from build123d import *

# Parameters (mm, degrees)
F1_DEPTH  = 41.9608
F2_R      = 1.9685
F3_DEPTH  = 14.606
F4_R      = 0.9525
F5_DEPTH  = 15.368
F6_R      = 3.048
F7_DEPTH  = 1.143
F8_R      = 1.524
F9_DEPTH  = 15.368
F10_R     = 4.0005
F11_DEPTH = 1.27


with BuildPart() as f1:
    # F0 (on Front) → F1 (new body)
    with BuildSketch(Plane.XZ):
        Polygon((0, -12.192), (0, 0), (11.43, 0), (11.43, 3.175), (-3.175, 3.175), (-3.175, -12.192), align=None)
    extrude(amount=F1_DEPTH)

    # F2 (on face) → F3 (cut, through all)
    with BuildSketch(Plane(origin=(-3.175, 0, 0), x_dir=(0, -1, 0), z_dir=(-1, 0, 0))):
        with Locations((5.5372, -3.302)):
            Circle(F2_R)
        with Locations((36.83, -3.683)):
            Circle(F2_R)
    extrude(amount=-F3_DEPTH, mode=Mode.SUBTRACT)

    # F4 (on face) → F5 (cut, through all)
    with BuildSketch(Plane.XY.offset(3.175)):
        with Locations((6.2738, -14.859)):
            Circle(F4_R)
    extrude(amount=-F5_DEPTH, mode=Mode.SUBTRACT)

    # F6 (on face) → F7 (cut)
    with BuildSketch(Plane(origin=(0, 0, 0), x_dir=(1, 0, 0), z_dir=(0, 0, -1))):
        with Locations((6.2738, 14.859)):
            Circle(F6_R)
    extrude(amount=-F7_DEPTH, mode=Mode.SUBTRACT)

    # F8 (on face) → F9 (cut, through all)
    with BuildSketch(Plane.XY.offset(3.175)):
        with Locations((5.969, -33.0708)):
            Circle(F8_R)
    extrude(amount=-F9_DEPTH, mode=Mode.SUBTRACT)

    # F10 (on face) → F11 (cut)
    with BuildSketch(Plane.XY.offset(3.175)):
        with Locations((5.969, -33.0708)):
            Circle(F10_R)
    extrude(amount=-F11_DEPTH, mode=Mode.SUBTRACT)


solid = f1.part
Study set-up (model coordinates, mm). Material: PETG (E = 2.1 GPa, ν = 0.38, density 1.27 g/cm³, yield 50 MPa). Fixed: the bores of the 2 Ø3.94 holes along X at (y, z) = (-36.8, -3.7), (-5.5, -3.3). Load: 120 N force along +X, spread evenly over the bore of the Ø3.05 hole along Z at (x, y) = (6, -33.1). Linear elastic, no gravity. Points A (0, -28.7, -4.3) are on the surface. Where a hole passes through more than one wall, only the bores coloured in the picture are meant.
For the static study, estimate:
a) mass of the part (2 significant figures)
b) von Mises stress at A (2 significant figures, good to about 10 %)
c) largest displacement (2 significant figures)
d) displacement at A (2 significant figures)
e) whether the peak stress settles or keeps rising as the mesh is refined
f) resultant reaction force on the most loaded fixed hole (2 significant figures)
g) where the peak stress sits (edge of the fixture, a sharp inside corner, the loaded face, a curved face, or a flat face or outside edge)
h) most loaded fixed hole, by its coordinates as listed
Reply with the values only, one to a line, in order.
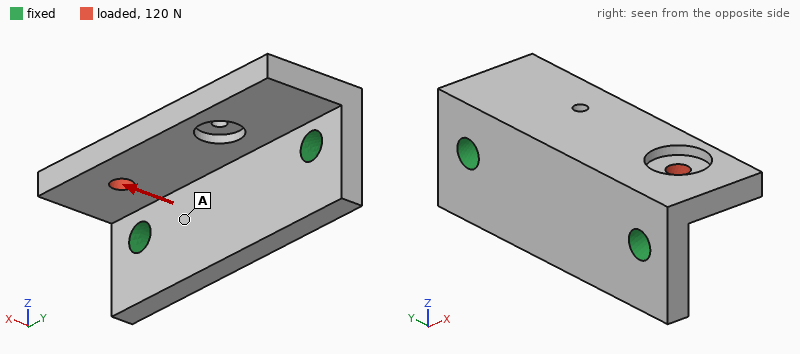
4.3 g
1.9 MPa
0.11 mm
0.018 mm
keeps rising
110 N
edge of the fixture
(-36.8, -3.7)
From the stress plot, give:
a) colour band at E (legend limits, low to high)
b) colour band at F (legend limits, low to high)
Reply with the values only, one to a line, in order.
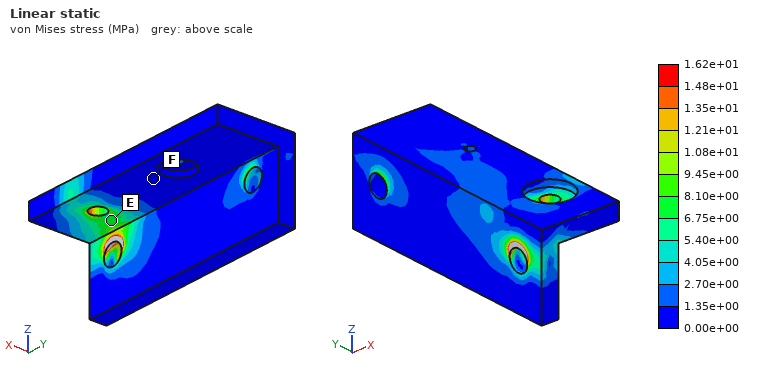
6.75e+00 to 8.10e+00 MPa
0.00e+00 to 1.35e+00 MPa
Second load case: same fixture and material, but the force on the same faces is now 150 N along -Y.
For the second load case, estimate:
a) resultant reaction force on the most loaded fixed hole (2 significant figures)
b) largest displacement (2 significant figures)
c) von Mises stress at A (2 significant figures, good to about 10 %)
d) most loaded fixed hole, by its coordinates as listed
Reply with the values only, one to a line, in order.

91 N
0.10 mm
1.7 MPa
(-36.8, -3.7)
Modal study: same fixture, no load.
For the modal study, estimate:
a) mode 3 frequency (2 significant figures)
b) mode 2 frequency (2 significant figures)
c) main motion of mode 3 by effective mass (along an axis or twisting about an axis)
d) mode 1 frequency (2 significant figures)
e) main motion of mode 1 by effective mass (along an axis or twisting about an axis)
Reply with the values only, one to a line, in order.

4700 Hz
3500 Hz
along X
2400 Hz
along Z
